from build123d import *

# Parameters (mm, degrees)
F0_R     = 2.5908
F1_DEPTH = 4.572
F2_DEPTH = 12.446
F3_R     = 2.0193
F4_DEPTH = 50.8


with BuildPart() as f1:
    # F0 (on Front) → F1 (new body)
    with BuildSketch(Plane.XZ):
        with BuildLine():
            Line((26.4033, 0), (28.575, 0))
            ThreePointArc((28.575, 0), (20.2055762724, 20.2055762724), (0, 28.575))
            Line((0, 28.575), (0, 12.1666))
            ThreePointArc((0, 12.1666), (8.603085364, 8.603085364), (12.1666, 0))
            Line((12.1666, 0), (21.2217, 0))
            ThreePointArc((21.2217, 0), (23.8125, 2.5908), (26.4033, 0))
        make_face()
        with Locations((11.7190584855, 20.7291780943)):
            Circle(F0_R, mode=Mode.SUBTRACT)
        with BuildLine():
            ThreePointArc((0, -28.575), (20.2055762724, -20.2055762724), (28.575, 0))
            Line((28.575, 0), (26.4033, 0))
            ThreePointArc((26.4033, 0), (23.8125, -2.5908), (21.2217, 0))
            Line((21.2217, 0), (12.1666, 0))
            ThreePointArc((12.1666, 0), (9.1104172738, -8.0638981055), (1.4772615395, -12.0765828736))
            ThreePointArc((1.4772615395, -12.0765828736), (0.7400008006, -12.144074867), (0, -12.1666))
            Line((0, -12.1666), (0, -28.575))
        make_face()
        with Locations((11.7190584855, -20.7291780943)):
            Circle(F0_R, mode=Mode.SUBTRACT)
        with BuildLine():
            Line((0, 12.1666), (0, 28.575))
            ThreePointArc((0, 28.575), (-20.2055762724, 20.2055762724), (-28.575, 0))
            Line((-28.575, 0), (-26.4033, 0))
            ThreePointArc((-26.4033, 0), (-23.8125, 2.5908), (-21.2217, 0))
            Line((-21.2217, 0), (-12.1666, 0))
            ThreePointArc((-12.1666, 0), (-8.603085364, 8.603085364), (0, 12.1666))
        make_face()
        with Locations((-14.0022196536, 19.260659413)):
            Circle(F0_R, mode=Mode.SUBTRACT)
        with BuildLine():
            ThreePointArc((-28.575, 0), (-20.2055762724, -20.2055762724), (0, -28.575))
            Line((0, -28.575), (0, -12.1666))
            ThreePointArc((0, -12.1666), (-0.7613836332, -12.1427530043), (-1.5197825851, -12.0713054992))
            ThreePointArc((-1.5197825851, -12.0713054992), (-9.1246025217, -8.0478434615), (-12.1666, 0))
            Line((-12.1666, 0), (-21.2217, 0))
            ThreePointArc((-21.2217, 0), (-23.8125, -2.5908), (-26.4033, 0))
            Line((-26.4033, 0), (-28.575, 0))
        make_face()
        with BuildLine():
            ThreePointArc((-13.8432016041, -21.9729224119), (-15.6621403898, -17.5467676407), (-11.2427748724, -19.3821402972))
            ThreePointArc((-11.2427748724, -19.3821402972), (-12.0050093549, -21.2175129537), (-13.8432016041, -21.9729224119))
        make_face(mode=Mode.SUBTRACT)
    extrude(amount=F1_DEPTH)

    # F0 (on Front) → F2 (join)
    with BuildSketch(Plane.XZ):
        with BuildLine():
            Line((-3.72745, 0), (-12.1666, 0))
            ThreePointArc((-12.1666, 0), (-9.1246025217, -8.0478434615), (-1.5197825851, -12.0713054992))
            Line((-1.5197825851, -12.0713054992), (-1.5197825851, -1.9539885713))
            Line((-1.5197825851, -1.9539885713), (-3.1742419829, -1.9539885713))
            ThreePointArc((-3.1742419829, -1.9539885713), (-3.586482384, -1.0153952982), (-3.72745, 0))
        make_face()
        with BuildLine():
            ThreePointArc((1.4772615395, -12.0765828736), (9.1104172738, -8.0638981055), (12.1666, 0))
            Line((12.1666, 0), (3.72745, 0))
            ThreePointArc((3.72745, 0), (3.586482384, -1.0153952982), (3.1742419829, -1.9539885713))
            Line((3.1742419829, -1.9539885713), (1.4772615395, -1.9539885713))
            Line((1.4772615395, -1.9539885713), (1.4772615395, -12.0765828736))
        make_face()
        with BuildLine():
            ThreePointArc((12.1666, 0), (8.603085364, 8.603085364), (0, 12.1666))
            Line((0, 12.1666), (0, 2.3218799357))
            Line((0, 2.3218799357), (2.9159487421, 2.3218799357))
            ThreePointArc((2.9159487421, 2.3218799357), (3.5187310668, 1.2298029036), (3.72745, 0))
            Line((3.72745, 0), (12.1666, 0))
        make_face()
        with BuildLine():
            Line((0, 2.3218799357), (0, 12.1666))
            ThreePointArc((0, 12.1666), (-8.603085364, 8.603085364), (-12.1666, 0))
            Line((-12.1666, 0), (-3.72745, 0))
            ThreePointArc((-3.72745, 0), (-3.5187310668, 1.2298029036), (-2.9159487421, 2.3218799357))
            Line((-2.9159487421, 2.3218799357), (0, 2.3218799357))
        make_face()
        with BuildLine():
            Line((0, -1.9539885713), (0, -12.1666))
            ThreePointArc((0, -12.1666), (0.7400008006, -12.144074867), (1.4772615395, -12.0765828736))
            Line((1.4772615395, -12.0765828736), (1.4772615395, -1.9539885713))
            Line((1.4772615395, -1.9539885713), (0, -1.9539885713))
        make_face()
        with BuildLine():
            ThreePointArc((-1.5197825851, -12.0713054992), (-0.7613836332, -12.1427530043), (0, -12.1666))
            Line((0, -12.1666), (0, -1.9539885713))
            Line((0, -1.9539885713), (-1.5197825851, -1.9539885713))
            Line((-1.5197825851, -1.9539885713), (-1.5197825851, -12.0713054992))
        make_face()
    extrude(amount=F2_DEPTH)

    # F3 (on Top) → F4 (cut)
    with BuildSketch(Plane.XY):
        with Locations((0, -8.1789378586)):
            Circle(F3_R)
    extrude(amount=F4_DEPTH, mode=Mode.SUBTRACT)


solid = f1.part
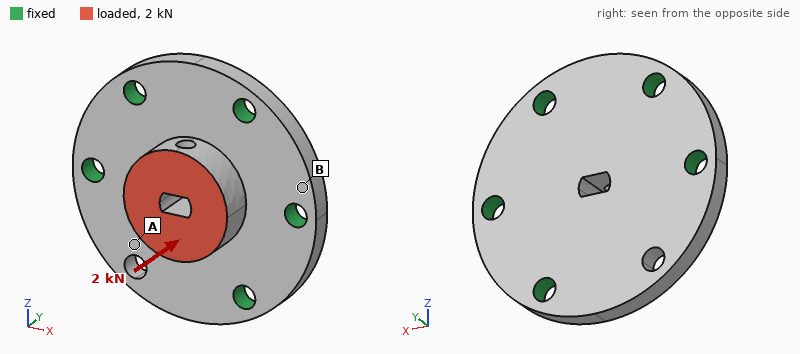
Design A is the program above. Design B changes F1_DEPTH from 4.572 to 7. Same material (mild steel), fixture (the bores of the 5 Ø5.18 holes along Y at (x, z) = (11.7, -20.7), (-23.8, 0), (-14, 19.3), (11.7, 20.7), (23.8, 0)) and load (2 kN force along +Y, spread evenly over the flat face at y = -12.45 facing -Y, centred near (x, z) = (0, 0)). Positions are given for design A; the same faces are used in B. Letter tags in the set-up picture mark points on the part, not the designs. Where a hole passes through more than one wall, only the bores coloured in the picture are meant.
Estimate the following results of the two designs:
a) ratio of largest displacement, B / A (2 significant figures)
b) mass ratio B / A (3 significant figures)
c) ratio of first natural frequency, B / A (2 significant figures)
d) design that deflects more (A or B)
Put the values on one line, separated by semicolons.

0.44; 1.33; 1.4; A
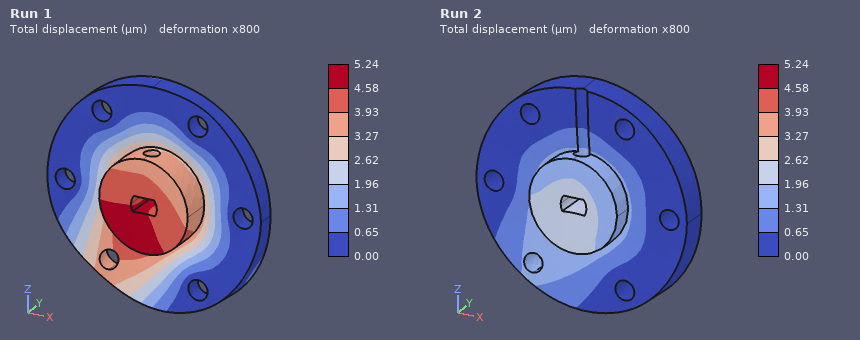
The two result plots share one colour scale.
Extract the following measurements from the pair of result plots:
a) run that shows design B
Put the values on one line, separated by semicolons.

Run 2
